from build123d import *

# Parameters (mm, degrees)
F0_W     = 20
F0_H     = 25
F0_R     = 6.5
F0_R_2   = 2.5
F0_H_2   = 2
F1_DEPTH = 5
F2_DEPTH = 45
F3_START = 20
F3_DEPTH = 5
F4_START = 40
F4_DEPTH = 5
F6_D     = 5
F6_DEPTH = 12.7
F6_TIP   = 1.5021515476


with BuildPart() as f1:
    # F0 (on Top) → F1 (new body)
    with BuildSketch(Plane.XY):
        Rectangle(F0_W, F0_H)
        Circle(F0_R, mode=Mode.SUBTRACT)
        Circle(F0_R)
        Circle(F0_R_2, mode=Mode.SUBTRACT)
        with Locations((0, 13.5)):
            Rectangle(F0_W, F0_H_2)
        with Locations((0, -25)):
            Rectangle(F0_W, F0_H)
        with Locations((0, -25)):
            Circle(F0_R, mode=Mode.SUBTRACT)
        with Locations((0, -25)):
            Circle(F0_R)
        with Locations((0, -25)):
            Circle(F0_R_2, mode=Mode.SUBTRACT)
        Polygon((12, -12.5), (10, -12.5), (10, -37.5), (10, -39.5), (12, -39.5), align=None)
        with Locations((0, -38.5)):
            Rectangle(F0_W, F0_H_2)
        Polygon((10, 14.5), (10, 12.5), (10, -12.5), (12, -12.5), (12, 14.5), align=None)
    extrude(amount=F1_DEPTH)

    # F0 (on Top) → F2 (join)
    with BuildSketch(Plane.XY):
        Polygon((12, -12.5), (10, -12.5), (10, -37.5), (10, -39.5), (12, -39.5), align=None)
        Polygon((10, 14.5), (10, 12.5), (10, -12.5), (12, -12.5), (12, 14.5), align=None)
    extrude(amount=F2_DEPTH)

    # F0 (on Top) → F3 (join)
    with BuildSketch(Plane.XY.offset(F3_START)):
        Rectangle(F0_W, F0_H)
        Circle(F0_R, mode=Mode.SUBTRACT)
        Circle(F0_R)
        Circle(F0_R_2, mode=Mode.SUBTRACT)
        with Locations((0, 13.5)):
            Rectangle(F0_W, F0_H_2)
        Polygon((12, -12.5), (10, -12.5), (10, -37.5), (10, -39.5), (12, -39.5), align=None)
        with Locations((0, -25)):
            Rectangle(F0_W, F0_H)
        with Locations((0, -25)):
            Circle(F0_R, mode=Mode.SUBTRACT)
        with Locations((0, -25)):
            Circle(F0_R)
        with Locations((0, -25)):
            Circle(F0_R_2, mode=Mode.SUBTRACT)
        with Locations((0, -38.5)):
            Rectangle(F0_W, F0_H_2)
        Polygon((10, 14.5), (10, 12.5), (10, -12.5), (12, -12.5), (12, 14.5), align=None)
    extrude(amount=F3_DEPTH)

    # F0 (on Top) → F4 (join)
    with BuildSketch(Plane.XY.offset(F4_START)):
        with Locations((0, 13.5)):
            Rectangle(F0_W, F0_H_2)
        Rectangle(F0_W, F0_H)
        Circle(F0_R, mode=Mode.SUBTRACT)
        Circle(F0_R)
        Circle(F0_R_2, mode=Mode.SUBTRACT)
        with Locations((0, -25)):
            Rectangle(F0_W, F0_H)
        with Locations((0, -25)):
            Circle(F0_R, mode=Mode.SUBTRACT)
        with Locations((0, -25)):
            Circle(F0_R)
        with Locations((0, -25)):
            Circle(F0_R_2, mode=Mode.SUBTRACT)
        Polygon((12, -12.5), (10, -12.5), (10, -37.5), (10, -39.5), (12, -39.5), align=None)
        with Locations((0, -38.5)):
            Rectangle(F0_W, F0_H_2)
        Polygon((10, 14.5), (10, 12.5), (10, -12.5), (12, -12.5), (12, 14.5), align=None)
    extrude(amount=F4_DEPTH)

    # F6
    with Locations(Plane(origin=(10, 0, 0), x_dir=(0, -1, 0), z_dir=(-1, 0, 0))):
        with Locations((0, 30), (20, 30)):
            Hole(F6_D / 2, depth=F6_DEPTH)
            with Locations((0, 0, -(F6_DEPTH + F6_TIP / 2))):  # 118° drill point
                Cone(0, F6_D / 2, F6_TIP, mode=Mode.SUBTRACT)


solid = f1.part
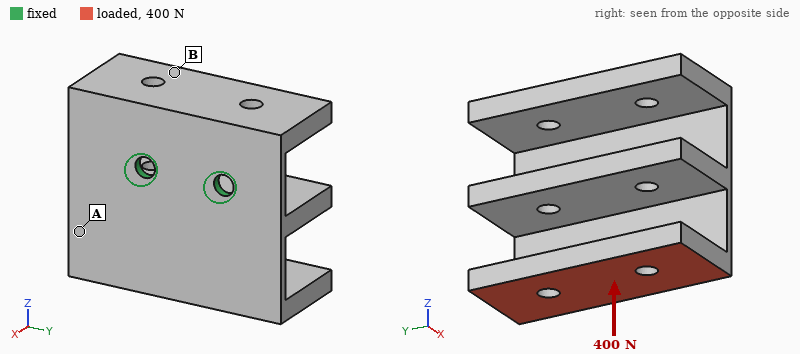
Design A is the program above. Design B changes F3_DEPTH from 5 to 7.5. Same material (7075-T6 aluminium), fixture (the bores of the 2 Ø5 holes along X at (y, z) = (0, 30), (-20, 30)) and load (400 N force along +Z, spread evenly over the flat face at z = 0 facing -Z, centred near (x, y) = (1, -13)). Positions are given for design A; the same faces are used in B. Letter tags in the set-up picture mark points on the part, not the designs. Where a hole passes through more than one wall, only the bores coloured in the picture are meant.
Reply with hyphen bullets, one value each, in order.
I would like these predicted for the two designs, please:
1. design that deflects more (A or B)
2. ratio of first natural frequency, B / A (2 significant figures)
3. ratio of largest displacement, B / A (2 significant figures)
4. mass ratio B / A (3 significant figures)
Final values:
- A
- 1.1
- 0.85
- 1.13
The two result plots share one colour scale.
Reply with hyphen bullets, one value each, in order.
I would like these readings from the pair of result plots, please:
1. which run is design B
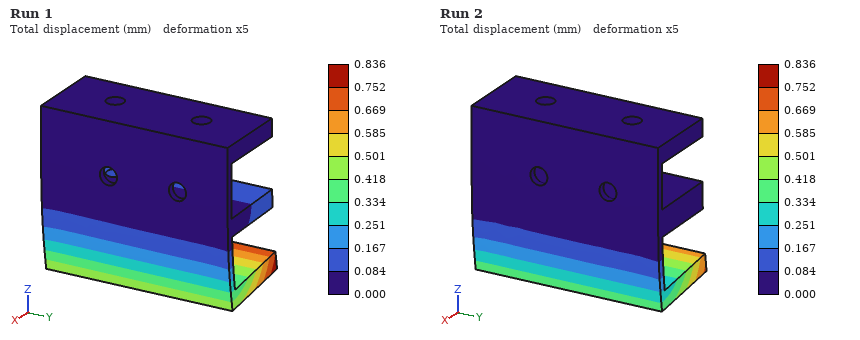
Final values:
- Run 2
